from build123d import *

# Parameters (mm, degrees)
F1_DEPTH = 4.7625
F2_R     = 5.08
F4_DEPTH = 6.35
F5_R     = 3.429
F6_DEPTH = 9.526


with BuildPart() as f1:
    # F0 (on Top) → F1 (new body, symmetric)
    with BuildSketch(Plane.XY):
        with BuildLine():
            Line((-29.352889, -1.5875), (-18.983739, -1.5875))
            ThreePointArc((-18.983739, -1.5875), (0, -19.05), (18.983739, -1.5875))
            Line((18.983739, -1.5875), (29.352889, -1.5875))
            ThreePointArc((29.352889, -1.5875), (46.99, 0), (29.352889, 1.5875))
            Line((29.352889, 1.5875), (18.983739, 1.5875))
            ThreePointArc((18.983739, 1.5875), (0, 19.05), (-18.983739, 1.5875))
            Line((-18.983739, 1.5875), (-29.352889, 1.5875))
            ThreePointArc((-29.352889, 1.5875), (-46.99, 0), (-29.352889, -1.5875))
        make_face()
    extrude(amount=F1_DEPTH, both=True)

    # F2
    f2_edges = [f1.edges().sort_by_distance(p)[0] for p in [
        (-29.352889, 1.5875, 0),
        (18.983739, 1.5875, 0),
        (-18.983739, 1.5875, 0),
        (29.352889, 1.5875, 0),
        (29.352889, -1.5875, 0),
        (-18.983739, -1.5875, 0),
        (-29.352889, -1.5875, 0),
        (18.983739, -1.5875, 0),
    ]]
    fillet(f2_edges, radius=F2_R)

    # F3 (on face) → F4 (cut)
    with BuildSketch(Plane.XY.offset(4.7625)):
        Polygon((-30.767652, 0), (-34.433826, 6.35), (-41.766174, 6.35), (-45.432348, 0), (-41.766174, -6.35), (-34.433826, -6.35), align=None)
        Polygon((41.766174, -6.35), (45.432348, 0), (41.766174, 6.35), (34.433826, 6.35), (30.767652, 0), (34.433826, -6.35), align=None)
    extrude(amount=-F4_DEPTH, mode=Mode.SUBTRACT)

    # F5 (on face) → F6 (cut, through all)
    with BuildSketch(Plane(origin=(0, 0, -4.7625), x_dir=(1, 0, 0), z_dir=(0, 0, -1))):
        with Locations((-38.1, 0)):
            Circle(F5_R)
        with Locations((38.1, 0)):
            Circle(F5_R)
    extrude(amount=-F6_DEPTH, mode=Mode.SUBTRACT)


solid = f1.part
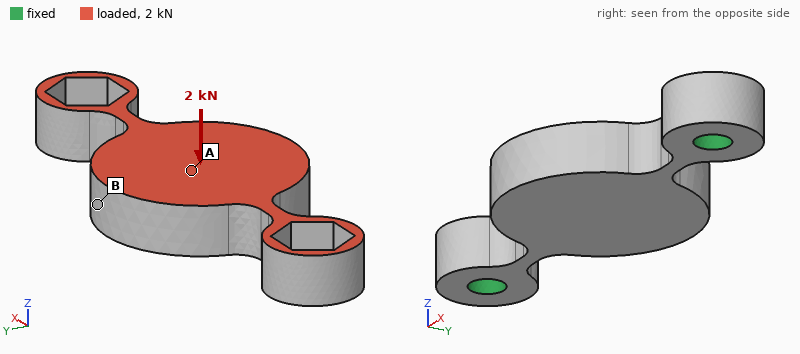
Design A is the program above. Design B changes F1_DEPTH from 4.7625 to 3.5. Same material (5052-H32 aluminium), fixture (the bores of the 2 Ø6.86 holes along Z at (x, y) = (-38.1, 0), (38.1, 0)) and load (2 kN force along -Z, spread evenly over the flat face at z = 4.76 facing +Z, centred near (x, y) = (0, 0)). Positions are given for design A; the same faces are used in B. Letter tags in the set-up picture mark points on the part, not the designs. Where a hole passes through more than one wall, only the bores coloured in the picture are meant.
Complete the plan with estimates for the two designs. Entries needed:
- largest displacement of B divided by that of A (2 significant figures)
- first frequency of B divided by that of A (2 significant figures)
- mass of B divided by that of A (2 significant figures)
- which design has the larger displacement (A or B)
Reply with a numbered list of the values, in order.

1. 2.3
2. 0.86
3. 0.73
4. B
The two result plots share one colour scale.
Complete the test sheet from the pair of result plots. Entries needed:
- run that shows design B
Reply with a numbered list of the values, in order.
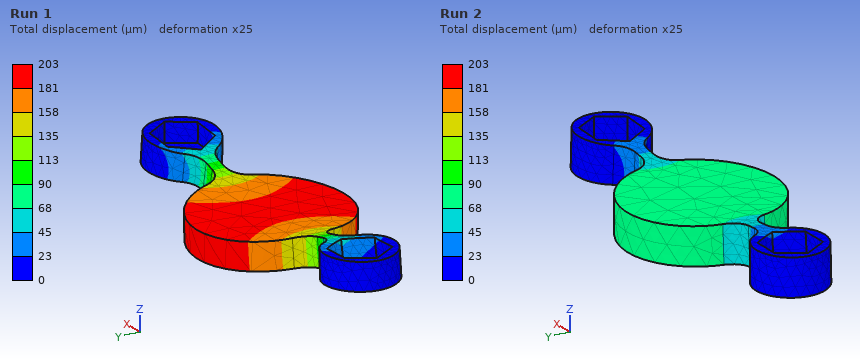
1. Run 1
